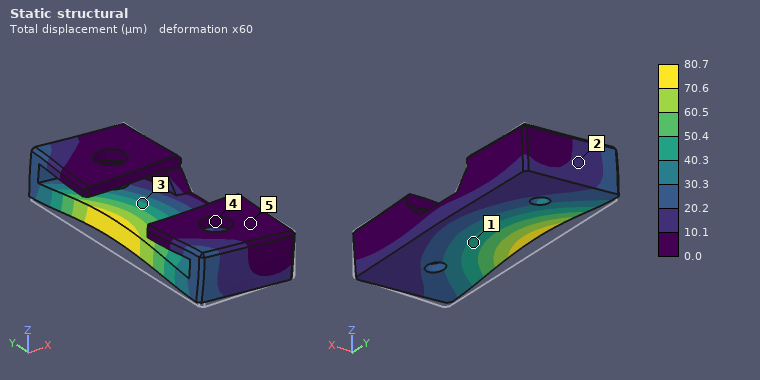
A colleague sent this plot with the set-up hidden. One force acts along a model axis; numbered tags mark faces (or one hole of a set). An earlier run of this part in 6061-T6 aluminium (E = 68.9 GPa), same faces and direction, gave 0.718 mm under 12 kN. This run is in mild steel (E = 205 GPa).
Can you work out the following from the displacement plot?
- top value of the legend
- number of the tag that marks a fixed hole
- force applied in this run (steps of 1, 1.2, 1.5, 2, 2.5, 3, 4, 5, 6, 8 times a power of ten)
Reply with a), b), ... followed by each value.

a) 80.7 µm
b) 4
c) 4 kN
